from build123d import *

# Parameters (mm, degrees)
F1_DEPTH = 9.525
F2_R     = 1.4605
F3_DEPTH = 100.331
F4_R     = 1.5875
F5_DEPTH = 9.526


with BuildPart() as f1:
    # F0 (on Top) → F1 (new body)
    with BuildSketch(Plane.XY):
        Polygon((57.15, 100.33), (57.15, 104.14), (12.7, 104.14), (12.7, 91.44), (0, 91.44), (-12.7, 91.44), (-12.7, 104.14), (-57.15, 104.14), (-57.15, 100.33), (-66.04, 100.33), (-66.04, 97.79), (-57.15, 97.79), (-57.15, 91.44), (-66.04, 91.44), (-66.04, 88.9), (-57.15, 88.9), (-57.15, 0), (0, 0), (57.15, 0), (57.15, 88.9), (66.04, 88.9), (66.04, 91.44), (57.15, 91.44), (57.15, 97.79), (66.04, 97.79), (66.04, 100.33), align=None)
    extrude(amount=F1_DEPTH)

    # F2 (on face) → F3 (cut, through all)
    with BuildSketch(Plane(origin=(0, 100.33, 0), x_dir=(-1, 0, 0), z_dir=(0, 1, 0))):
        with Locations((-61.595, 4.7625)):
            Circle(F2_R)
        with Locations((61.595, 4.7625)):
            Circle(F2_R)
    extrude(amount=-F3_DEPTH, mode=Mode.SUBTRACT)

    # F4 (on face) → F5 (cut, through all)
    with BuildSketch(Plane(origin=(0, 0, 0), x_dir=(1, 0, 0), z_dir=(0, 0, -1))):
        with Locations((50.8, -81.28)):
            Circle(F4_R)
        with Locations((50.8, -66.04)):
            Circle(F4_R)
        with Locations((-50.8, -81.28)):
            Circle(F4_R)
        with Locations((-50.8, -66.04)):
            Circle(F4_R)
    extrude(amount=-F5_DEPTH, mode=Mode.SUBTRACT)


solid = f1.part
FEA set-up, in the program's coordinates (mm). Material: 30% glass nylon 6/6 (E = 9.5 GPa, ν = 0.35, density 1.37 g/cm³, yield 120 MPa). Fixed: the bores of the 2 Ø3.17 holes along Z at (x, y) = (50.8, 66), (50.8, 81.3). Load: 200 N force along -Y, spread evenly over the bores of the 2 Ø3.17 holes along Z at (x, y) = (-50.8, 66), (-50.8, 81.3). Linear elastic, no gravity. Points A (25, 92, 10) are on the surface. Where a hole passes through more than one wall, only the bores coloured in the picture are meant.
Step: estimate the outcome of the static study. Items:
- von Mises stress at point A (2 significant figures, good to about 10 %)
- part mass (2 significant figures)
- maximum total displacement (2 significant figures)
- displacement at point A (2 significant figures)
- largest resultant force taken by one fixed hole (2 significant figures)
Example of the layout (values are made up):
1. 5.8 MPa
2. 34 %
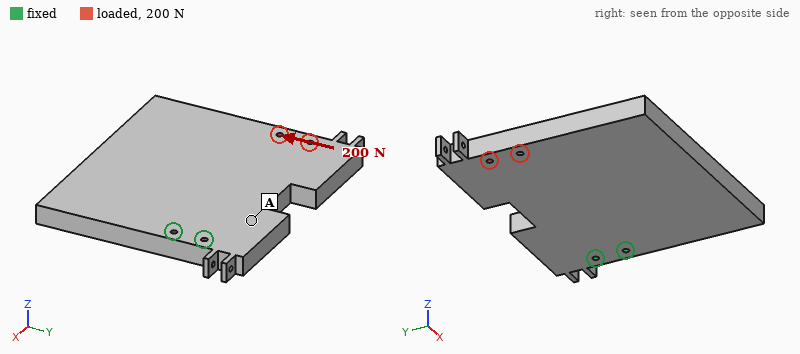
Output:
1. 2.2 MPa
2. 150 g
3. 0.26 mm
4. 0.056 mm
5. 1.2 kN
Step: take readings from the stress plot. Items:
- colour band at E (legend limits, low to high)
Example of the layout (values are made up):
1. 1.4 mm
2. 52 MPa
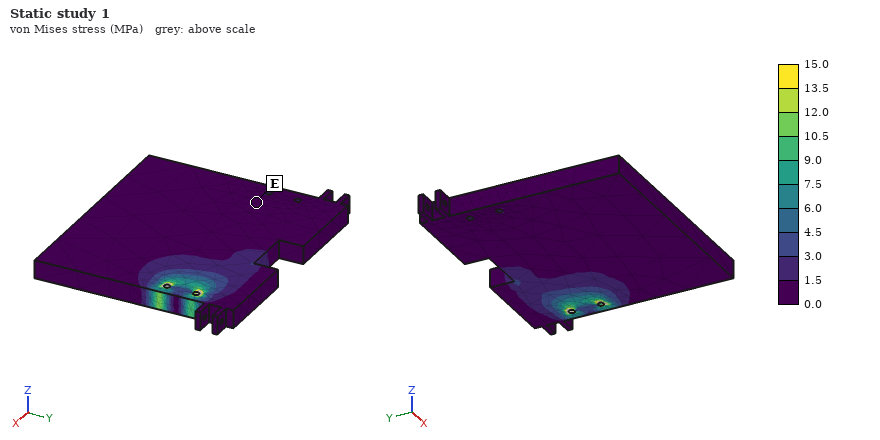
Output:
1. 0.0 to 1.5 MPa
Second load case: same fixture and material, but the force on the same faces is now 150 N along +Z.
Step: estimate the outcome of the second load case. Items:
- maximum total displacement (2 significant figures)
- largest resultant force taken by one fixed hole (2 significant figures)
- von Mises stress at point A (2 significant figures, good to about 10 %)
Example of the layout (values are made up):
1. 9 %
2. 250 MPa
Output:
1. 1.7 mm
2. 76 N
3. 9.6 MPa
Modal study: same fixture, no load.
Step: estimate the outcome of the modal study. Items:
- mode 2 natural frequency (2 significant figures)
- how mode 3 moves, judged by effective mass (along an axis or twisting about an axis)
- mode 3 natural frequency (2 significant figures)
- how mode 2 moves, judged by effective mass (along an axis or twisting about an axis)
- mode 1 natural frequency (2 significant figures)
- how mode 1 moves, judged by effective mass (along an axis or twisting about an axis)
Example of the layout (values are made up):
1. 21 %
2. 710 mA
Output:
1. 500 Hz
2. along Y
3. 590 Hz
4. twisting about X
5. 240 Hz
6. along Z
